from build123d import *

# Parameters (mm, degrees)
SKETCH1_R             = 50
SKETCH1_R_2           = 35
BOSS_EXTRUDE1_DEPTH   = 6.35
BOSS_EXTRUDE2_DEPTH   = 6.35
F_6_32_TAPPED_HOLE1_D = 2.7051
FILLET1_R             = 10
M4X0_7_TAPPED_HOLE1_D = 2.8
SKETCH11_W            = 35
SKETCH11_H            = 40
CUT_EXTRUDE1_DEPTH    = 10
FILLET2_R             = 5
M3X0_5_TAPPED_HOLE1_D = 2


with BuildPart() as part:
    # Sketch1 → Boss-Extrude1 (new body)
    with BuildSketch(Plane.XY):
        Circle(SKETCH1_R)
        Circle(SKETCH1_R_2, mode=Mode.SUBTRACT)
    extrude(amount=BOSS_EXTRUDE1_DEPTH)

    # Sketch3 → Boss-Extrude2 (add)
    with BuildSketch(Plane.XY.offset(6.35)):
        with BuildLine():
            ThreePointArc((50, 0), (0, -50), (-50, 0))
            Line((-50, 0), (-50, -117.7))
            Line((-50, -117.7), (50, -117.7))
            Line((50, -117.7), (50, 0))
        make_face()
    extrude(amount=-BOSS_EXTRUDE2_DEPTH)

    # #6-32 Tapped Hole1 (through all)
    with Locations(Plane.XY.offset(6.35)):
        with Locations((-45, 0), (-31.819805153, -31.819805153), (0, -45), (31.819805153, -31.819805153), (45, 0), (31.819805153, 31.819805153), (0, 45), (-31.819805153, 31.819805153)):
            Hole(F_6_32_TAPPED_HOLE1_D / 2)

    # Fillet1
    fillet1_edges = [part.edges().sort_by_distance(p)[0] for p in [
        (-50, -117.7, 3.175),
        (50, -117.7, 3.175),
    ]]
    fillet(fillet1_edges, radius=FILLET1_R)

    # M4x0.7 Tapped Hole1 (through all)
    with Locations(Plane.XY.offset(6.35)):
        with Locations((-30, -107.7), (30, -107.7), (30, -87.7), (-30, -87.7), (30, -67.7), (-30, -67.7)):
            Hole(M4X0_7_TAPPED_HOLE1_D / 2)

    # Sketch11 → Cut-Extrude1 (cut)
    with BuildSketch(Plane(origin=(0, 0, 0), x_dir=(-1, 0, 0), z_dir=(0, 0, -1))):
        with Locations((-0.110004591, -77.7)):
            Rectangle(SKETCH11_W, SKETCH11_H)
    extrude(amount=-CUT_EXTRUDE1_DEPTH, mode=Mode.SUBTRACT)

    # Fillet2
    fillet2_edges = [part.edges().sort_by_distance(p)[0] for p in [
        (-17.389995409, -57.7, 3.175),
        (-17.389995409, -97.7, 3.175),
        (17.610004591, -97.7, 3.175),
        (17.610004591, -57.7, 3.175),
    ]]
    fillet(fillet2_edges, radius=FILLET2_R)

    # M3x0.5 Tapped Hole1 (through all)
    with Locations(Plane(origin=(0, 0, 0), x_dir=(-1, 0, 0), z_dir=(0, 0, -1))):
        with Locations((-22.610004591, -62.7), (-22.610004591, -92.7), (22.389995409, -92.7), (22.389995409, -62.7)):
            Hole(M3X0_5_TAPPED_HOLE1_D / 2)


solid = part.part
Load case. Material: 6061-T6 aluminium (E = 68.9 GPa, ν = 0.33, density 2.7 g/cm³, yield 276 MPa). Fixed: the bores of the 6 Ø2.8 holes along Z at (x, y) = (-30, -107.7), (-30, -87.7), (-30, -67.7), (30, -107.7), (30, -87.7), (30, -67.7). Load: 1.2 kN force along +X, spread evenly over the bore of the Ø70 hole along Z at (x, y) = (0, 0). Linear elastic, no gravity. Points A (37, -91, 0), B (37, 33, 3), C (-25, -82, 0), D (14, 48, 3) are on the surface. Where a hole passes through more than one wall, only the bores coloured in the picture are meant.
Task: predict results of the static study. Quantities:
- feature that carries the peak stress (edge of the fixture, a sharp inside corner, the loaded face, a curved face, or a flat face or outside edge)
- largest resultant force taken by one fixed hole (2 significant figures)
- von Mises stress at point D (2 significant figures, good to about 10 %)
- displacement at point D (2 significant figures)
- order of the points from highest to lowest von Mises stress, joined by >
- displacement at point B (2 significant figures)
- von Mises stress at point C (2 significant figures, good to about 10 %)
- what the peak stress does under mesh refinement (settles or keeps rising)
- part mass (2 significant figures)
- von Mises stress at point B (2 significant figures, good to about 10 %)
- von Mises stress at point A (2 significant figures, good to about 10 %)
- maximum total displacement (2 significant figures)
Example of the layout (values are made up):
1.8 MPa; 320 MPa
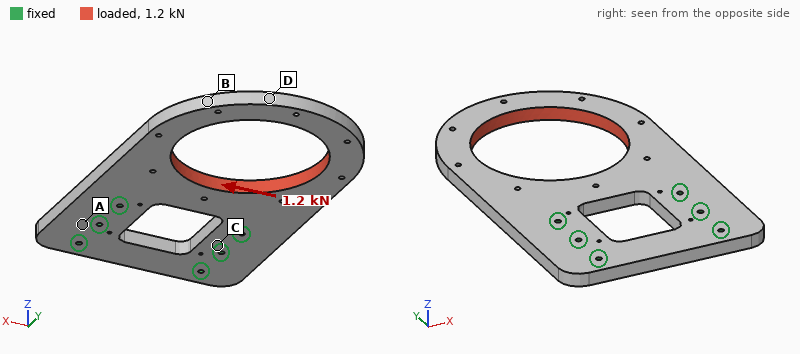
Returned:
edge of the fixture; 1.1 kN; 6.9 MPa; 73 µm; B > D > A > C; 74 µm; 1.9 MPa; keeps rising; 180 g; 14 MPa; 3.9 MPa; 75 µm
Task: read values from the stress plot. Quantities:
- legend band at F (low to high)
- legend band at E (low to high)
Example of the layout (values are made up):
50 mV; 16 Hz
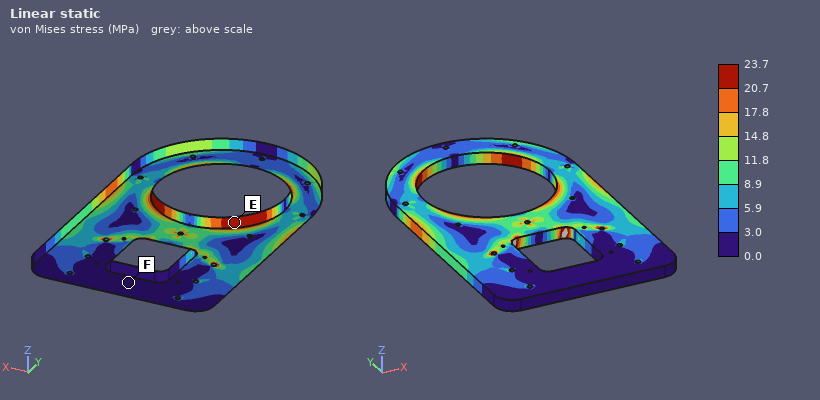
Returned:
0.0 to 3.0 MPa; 20.7 to 23.7 MPa
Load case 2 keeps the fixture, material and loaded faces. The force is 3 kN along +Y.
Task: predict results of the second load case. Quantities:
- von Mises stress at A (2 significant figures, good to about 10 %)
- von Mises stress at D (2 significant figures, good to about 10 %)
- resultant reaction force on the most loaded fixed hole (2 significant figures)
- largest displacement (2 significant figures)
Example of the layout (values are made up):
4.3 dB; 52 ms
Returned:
3.0 MPa; 13 MPa; 980 N; 32 µm
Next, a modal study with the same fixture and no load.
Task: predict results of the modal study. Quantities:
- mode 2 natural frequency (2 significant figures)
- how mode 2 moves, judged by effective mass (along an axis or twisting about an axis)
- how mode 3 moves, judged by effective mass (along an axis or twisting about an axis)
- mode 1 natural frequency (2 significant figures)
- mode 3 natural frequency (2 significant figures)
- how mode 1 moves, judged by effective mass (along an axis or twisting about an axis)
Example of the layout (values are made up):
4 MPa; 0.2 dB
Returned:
1100 Hz; twisting about Y; along Z; 420 Hz; 2000 Hz; along Z
